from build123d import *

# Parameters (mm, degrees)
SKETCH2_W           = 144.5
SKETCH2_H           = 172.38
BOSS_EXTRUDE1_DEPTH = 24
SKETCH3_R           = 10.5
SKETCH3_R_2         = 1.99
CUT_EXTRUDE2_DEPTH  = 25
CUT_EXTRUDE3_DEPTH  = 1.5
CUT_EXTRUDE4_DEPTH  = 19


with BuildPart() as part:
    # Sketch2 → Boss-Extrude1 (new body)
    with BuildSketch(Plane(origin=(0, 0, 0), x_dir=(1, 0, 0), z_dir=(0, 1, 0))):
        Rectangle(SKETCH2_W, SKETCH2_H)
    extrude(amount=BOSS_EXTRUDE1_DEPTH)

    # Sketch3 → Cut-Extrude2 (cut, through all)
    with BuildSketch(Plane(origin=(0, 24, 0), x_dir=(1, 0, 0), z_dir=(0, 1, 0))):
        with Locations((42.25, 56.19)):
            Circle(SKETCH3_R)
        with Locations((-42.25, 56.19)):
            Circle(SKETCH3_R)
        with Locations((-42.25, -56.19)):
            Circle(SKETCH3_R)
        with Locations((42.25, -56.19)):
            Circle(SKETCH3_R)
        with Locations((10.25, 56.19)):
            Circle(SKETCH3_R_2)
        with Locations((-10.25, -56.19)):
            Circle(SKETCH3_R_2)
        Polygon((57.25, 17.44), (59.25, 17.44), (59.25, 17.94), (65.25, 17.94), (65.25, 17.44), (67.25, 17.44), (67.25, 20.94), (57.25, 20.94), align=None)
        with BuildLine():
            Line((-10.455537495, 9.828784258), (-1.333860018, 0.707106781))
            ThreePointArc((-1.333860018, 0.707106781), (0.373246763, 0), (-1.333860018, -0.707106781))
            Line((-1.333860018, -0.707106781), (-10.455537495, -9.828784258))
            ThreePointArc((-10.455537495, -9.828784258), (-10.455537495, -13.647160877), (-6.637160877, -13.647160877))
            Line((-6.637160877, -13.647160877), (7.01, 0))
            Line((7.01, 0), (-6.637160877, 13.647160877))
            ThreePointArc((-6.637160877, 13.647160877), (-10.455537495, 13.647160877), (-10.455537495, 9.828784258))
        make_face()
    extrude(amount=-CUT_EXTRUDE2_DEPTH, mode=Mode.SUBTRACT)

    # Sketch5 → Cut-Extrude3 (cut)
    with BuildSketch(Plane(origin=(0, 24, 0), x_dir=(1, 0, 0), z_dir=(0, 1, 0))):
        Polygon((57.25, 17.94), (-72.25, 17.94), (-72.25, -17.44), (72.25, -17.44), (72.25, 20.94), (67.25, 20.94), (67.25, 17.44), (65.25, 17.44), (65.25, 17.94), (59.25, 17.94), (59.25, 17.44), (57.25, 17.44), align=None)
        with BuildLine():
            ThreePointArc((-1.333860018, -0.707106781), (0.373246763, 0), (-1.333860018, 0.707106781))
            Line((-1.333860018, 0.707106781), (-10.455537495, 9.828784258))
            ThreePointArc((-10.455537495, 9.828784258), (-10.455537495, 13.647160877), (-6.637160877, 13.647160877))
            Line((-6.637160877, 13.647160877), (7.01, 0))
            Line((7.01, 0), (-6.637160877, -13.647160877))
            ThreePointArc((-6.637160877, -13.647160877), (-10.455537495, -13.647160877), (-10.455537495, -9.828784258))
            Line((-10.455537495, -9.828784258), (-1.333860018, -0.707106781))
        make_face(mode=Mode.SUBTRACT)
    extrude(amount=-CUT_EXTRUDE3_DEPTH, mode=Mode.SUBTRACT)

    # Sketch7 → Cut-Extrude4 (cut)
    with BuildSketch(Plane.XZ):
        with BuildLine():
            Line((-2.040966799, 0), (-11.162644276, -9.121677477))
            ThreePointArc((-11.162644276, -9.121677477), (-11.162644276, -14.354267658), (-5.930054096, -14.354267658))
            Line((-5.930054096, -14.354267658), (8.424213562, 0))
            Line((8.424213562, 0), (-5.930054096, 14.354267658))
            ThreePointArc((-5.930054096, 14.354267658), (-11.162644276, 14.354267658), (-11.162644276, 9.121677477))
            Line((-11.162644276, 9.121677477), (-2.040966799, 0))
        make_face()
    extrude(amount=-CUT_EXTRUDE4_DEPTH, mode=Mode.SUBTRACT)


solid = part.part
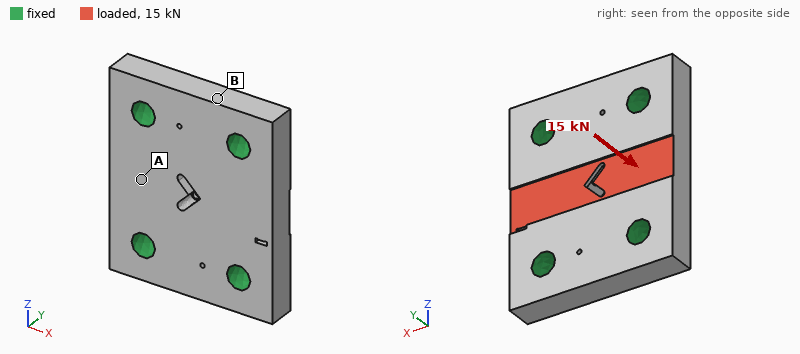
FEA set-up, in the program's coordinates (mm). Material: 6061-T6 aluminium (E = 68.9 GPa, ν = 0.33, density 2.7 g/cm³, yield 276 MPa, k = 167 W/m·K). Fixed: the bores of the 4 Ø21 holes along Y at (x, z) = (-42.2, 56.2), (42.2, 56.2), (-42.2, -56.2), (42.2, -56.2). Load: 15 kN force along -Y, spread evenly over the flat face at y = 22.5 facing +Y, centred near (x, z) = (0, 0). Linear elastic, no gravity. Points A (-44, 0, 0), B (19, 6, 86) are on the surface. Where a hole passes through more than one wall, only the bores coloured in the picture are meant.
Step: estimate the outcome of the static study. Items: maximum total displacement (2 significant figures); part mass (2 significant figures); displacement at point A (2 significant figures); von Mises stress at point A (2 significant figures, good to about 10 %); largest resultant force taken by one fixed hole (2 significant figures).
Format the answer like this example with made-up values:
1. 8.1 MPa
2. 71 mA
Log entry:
1. 19 µm
2. 1.5 kg
3. 12 µm
4. 11 MPa
5. 3.8 kN
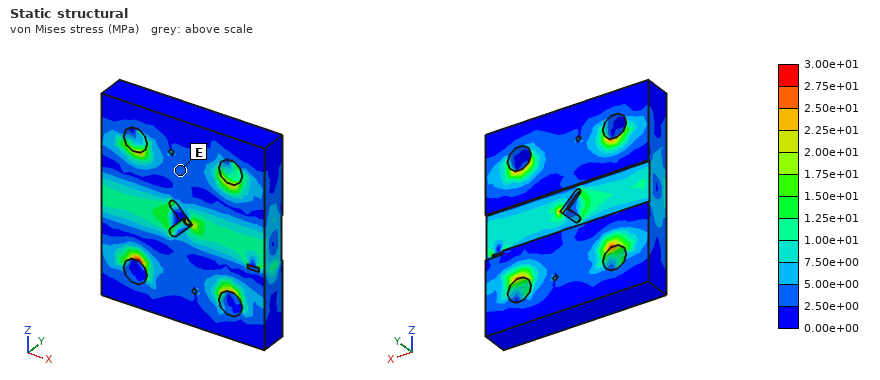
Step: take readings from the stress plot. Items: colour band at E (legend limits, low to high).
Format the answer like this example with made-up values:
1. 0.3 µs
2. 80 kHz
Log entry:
1. 2.50e+00 to 5.00e+00 MPa
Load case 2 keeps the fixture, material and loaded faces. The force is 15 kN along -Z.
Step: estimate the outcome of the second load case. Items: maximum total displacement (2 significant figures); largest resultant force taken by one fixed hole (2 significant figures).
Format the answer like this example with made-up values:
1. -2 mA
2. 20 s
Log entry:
1. 5.0 µm
2. 4.0 kN
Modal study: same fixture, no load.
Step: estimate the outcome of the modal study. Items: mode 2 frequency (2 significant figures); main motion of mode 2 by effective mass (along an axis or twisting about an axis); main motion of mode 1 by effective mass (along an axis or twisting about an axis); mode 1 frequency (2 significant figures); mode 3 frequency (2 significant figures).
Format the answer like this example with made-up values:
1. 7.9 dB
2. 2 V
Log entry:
1. 9200 Hz
2. twisting about Z
3. along Y
4. 8100 Hz
5. 10 kHz
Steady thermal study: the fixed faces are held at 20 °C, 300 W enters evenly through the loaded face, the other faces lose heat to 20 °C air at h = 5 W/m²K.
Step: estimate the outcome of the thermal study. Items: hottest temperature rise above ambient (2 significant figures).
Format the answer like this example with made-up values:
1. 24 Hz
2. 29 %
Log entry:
1. 17 K
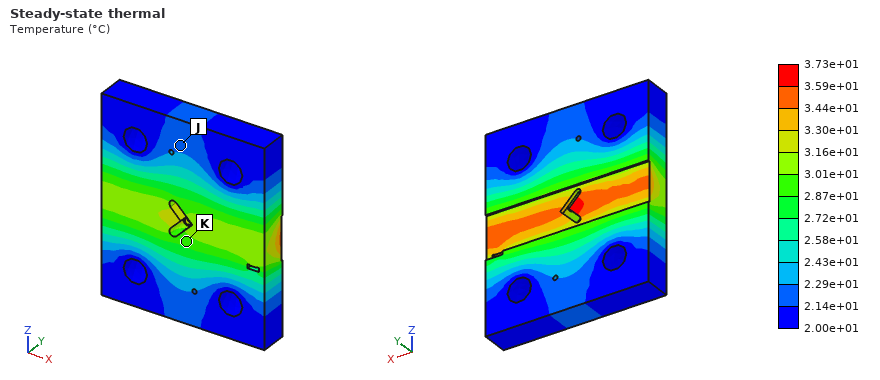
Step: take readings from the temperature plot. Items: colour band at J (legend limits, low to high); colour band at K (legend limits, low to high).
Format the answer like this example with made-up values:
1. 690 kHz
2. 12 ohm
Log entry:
1. 2.14e+01 to 2.29e+01 °C
2. 2.87e+01 to 3.01e+01 °C
